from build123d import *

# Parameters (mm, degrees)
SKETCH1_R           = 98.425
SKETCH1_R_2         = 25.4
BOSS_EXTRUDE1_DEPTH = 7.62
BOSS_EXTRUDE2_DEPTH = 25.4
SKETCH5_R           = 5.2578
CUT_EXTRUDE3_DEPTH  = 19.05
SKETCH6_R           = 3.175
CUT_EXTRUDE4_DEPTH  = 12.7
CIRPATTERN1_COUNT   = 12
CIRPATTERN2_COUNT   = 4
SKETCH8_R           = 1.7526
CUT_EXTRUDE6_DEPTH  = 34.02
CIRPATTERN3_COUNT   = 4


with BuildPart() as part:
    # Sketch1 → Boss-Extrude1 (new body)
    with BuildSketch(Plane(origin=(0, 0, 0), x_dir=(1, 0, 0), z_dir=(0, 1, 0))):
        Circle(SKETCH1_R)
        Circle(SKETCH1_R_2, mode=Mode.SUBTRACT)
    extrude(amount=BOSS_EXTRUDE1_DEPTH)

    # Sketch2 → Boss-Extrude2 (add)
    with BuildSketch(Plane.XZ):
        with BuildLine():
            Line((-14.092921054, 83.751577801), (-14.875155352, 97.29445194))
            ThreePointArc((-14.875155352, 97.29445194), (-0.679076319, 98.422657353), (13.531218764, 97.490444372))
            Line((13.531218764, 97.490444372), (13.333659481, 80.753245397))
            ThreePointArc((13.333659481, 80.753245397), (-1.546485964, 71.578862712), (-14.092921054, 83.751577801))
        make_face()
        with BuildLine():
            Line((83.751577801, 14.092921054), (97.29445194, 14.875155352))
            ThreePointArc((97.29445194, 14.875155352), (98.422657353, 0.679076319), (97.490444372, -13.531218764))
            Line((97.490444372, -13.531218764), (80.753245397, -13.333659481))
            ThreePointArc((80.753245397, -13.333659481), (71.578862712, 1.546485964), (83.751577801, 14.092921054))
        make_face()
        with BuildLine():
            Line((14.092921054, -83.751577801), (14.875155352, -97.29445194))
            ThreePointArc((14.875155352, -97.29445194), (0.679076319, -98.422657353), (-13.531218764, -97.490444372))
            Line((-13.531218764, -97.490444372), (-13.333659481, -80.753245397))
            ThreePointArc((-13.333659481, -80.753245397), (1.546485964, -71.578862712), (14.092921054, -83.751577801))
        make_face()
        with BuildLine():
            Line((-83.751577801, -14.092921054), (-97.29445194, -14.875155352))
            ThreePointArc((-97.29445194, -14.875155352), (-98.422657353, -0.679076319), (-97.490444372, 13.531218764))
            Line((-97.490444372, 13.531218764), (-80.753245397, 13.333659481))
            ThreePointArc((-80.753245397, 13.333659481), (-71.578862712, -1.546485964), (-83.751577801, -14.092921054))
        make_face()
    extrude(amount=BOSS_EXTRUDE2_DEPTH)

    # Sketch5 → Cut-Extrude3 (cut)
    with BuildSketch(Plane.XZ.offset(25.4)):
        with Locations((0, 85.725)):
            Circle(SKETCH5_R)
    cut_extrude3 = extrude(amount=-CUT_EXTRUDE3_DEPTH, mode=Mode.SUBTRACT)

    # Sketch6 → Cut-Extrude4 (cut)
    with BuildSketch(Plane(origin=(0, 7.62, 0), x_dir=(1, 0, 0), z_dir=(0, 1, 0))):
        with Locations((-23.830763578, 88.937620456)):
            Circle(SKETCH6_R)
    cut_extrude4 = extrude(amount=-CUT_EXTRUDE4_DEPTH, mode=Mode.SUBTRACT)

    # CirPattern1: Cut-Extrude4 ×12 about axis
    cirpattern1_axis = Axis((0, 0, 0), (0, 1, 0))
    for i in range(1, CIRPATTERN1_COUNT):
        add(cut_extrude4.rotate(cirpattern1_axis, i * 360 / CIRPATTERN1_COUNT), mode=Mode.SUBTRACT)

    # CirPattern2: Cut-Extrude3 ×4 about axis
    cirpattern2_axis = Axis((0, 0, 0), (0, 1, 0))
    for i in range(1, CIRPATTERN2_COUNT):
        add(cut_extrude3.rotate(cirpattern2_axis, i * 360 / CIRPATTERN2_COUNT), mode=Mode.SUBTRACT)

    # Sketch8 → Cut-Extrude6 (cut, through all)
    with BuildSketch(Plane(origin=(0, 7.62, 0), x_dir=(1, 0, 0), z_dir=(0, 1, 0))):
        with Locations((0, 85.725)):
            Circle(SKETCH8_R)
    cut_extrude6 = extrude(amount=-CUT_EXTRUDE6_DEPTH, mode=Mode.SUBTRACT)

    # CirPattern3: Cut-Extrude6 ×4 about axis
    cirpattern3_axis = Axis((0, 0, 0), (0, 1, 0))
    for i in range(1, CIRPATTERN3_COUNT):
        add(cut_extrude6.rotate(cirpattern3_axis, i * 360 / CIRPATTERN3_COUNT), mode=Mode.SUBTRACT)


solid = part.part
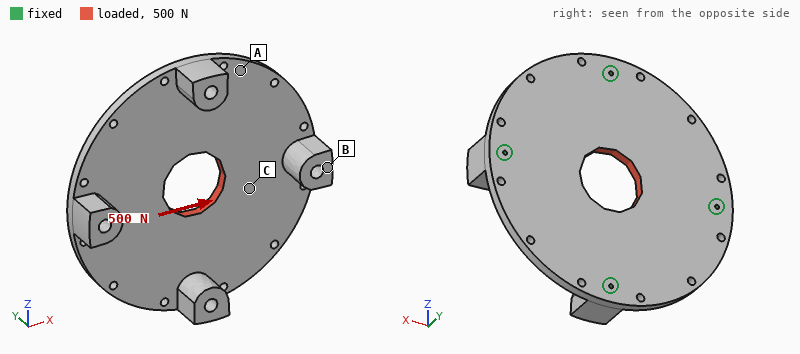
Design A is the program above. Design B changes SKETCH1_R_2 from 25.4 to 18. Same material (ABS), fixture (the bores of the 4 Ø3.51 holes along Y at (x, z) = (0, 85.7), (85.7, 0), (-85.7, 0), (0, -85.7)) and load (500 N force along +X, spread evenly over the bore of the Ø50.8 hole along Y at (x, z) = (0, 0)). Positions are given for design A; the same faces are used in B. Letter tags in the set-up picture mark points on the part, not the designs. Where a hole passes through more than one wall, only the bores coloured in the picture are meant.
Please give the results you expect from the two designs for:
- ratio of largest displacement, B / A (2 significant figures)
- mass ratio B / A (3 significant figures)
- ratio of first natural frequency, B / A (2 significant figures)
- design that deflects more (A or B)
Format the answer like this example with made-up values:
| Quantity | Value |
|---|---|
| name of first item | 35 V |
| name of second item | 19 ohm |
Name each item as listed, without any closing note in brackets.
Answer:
| Quantity | Value |
|---|---|
| ratio of largest displacement, B / A | 1.1 |
| mass ratio B / A | 1.03 |
| ratio of first natural frequency, B / A | 0.94 |
| design that deflects more | B |
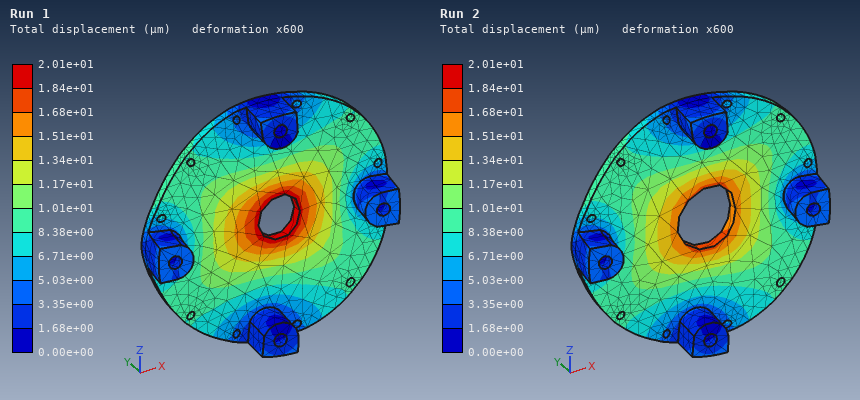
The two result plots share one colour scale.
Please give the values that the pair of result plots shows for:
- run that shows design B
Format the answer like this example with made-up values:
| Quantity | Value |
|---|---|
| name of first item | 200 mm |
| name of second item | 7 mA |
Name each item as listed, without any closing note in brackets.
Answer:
| Quantity | Value |
|---|---|
| run that shows design B | Run 1 |
